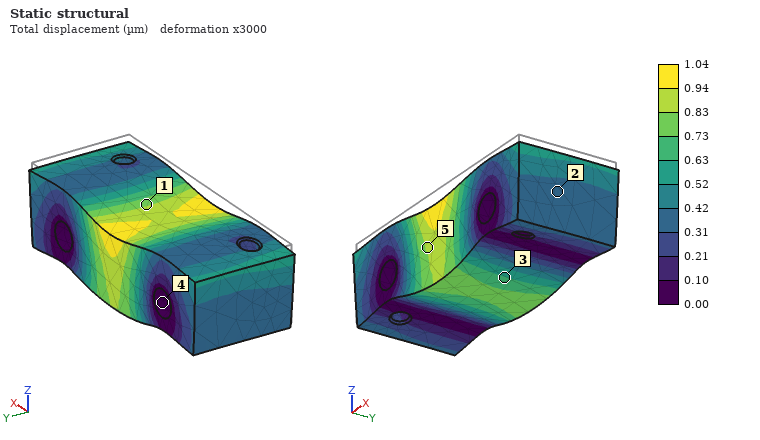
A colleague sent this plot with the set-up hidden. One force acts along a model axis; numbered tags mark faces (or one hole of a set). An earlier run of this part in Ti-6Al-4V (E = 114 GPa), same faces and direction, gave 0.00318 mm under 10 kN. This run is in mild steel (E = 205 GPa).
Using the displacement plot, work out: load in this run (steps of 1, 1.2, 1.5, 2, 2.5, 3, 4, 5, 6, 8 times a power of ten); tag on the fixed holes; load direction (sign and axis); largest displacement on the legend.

6 kN
4
-Z
1.04 µm
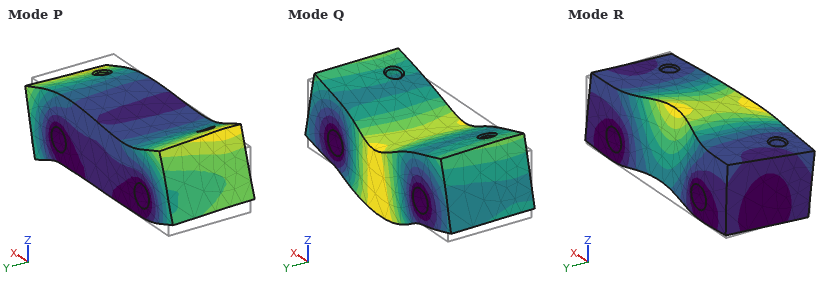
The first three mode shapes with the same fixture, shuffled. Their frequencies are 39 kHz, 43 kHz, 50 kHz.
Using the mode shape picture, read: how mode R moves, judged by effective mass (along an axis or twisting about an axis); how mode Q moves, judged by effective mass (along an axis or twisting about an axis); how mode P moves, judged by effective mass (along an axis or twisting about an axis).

along Y
along Z
along X
